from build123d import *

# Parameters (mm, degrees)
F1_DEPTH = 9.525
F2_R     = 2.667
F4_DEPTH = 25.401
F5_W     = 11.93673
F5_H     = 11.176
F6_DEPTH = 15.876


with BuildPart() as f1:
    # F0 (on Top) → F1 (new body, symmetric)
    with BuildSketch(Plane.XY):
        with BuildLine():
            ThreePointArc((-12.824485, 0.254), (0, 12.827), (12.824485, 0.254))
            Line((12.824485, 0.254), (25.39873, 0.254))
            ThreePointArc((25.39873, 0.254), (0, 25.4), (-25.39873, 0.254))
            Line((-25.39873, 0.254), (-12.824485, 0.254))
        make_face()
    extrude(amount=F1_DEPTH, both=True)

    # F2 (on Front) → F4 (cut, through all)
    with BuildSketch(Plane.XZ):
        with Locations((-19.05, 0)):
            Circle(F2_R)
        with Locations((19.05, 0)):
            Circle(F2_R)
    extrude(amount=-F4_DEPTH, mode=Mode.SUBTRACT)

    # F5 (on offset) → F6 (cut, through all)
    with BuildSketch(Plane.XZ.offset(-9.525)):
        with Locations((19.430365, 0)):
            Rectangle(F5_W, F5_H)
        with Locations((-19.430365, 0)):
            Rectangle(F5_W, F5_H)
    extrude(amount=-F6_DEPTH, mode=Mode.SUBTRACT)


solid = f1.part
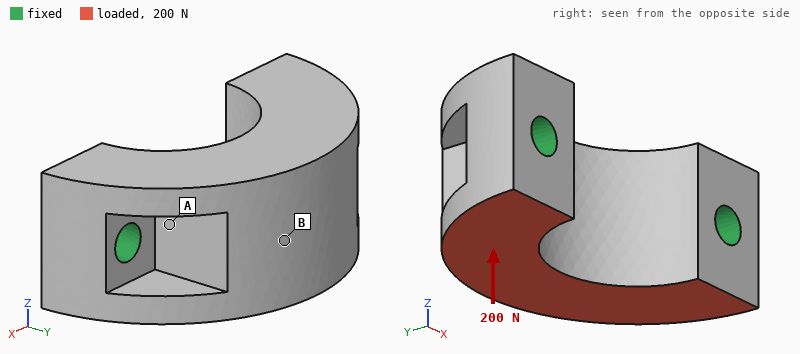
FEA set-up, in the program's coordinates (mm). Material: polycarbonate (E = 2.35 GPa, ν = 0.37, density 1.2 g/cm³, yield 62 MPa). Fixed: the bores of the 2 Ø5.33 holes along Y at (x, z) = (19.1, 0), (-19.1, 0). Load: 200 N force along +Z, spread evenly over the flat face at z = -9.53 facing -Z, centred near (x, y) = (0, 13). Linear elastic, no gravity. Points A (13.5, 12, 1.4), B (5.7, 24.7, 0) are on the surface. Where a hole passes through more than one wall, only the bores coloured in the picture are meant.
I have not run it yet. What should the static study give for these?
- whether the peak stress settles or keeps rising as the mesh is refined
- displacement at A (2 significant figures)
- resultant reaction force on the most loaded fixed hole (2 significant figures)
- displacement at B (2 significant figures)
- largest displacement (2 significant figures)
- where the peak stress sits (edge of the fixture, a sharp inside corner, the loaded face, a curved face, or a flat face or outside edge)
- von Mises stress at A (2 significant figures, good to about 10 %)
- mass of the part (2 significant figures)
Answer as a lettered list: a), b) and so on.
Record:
a) keeps rising
b) 17 µm
c) 100 N
d) 43 µm
e) 49 µm
f) edge of the fixture
g) 1.6 MPa
h) 15 g
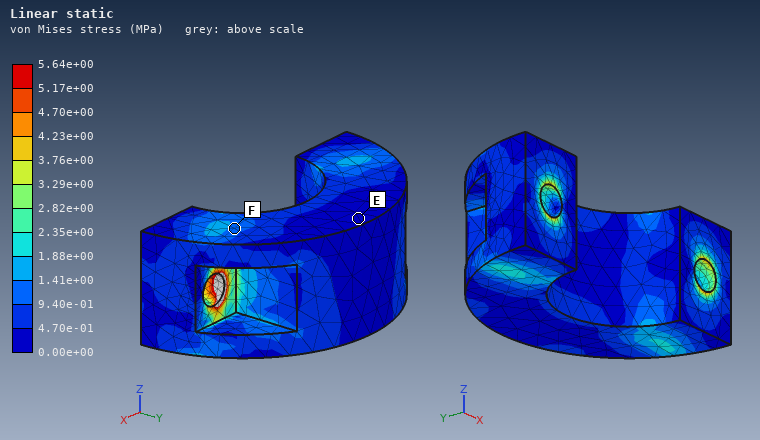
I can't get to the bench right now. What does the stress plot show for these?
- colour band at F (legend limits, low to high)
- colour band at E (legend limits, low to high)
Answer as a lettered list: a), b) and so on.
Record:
a) 9.40e-01 to 1.41e+00 MPa
b) 0.00e+00 to 4.70e-01 MPa
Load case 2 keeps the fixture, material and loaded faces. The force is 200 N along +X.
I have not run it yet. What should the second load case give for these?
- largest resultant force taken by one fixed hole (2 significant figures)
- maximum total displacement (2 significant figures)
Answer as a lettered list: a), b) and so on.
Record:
a) 110 N
b) 21 µm
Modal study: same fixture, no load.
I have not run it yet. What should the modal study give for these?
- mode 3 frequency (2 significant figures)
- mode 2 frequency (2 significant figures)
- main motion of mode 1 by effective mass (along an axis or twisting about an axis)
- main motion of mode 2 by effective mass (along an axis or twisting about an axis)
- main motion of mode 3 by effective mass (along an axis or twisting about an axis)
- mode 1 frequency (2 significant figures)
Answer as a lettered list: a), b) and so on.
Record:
a) 7500 Hz
b) 7000 Hz
c) along Z
d) along X
e) along Y
f) 3100 Hz
